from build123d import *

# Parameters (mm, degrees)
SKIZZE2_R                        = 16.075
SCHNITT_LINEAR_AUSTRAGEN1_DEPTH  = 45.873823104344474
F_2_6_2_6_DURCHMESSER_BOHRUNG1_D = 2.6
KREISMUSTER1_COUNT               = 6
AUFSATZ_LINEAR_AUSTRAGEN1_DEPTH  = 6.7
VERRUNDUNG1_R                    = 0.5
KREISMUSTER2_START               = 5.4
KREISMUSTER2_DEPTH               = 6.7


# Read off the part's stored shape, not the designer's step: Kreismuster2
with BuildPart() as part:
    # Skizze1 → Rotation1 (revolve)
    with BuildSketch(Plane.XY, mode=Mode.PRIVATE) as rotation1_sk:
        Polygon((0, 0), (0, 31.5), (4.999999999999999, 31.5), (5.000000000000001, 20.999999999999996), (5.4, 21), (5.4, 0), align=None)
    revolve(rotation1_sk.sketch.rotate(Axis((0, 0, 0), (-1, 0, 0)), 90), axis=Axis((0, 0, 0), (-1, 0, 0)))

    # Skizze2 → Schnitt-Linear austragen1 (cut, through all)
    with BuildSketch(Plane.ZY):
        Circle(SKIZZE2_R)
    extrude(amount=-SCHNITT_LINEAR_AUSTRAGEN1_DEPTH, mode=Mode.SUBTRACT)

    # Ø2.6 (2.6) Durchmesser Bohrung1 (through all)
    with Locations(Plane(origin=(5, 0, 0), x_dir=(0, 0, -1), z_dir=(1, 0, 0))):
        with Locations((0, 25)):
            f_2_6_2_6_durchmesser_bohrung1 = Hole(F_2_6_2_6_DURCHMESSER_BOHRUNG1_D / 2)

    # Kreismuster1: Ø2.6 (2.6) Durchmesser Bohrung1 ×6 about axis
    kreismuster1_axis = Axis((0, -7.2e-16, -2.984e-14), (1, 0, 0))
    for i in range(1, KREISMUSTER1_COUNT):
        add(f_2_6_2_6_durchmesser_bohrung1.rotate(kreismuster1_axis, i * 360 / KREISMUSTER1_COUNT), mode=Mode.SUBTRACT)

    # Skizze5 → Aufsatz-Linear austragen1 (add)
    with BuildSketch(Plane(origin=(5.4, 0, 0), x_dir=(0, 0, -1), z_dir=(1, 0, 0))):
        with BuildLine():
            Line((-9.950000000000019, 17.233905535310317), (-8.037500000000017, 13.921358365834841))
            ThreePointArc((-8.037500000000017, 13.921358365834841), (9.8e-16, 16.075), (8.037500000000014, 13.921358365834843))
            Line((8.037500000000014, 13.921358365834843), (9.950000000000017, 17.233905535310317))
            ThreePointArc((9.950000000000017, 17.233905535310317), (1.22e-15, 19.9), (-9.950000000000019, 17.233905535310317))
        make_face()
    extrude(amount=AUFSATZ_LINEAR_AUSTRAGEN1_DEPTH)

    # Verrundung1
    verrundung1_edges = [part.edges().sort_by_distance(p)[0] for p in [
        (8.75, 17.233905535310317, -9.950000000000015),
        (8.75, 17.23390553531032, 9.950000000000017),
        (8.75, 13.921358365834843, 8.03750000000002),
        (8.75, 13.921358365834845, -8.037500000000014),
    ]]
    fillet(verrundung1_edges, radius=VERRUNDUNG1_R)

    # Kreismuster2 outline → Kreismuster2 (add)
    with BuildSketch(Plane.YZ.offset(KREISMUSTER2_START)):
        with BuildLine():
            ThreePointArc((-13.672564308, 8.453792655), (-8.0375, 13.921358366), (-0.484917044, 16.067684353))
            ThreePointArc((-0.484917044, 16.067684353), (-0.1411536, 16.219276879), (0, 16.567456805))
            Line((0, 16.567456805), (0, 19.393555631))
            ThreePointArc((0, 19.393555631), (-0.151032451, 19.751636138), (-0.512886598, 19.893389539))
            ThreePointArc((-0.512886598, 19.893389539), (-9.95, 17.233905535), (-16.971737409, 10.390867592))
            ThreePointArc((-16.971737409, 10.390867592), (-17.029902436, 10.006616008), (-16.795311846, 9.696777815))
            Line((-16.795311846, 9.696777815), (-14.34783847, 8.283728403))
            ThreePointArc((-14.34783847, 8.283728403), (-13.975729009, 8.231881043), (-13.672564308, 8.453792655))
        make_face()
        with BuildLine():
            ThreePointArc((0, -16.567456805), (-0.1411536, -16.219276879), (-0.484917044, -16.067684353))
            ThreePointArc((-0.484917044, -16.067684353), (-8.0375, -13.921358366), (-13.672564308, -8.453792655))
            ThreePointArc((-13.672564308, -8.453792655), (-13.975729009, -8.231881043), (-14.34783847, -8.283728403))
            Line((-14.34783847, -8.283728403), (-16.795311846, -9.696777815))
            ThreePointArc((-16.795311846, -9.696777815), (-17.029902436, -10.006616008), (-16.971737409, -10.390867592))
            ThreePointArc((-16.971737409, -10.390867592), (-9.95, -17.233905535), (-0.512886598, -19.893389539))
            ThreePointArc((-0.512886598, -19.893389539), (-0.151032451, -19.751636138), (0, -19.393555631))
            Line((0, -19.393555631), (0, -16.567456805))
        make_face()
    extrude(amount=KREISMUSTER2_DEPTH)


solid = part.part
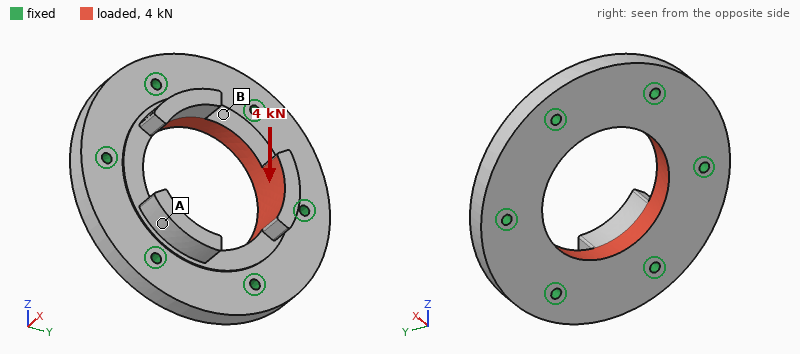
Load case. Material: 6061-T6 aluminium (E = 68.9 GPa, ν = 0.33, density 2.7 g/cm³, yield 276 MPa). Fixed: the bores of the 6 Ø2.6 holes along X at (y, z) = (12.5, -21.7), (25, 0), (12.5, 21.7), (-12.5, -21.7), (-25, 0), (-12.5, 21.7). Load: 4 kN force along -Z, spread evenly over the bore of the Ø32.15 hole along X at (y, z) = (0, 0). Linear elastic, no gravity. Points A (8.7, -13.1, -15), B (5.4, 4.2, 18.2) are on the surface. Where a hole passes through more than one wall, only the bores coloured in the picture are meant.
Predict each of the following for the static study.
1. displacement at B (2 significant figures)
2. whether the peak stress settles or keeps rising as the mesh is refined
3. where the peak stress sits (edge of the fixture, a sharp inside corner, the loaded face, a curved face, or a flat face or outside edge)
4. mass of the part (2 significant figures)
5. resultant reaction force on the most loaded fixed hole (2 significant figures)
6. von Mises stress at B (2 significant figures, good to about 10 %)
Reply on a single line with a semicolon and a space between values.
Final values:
1.7 µm; keeps rising; a sharp inside corner; 35 g; 810 N; 6.9 MPa
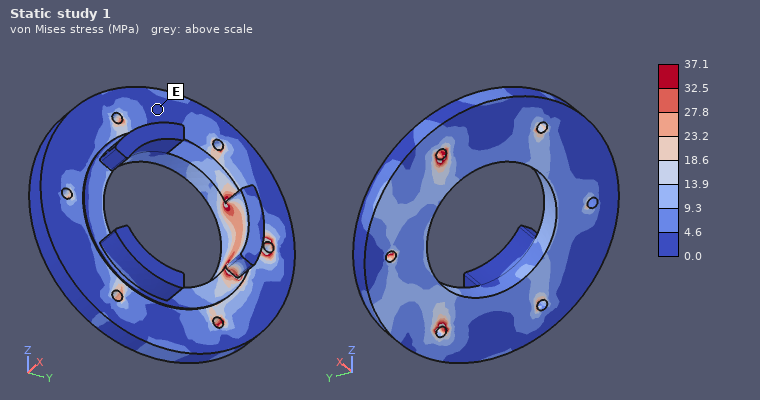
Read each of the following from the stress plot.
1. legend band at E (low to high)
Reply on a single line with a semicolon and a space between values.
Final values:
0.0 to 4.6 MPa
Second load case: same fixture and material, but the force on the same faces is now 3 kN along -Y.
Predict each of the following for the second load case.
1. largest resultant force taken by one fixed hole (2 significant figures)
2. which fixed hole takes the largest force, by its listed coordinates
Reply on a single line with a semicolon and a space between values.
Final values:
900 N; (25, 0)
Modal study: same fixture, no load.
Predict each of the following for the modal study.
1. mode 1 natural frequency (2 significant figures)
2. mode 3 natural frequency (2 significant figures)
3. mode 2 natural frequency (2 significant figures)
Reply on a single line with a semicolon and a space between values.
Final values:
22 kHz; 25 kHz; 23 kHz
